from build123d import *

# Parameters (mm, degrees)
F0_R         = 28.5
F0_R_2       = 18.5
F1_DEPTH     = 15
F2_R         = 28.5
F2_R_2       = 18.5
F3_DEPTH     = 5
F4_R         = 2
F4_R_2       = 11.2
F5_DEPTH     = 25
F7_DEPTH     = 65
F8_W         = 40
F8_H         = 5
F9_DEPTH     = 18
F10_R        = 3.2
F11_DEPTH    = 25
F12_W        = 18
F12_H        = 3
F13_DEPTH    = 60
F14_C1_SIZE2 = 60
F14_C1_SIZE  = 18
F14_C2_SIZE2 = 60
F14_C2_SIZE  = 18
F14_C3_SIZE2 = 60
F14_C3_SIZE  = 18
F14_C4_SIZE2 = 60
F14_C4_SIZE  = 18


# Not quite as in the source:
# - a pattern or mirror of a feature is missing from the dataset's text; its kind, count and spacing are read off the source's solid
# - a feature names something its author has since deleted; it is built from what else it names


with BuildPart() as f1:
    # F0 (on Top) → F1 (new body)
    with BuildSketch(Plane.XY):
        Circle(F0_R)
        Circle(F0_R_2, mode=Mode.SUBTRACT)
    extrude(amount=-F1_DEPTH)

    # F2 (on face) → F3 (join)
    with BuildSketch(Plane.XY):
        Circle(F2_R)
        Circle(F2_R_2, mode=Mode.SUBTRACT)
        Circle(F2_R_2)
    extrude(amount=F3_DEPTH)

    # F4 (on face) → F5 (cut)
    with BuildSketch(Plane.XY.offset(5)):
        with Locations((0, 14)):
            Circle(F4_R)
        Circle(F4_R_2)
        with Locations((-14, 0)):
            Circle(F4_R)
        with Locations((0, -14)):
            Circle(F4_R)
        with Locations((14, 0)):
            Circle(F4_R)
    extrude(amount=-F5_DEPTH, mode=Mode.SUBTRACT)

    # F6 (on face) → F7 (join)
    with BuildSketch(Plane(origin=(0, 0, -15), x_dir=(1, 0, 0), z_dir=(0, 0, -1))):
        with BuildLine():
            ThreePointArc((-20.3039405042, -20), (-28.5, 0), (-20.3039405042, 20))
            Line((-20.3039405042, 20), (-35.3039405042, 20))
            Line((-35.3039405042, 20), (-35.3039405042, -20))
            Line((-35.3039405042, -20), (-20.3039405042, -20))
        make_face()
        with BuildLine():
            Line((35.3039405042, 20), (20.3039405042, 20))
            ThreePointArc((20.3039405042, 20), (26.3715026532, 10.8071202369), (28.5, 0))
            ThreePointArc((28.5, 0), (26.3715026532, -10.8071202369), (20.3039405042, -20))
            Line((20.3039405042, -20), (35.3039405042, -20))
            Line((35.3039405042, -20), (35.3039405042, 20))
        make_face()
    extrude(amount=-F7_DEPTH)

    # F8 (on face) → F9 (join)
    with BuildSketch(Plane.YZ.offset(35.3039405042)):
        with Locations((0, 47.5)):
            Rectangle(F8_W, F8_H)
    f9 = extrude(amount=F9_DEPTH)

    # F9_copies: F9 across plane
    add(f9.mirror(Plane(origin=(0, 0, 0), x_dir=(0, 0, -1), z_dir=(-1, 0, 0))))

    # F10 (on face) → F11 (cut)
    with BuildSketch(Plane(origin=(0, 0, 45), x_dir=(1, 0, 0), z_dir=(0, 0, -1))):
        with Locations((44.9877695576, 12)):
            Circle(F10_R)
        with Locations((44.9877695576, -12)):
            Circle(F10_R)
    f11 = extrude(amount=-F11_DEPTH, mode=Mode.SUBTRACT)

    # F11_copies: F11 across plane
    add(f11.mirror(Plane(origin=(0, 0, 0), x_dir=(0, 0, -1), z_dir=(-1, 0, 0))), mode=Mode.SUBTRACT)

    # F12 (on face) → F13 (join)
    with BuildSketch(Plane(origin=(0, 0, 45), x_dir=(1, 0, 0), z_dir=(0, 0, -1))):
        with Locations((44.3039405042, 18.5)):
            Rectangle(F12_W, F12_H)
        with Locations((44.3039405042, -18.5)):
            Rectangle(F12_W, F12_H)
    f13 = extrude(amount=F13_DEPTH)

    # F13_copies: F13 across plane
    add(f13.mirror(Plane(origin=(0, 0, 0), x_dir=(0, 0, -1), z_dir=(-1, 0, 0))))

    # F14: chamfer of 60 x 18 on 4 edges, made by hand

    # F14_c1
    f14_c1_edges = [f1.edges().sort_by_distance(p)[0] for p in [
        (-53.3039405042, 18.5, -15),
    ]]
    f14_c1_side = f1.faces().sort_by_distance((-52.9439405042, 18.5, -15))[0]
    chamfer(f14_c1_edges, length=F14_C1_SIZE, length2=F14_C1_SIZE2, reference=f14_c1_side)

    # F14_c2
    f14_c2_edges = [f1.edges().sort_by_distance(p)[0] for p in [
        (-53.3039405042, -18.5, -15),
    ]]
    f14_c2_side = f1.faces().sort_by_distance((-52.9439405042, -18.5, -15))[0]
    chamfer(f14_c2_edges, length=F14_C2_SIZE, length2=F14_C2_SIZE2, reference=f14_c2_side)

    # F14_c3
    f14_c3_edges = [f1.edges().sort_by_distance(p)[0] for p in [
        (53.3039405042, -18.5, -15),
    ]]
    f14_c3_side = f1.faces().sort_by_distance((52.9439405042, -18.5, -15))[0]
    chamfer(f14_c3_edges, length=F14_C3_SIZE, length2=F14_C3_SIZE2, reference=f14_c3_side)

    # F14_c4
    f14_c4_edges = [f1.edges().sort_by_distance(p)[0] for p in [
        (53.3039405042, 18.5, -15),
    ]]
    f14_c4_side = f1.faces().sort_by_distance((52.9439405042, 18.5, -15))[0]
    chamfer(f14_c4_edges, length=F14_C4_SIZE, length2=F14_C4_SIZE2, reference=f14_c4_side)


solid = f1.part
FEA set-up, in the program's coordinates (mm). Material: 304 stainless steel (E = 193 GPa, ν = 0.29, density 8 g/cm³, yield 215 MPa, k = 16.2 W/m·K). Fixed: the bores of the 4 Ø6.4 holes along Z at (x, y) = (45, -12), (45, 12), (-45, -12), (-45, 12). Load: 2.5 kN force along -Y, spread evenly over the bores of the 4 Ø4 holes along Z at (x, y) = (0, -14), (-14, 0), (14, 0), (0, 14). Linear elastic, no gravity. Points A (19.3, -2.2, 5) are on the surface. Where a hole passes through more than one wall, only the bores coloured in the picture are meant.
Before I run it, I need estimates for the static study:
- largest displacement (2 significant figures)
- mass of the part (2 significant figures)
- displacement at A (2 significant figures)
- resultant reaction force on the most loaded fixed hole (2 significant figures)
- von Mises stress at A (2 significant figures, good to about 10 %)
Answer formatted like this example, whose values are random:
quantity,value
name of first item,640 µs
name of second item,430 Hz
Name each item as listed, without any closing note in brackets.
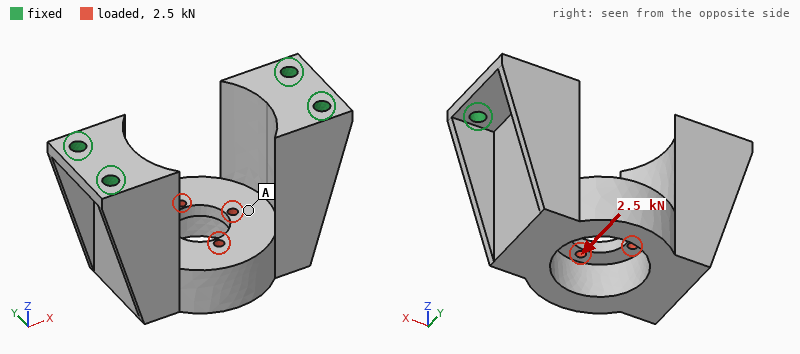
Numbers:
quantity,value
largest displacement,26 µm
mass of the part,760 g
displacement at A,18 µm
resultant reaction force on the most loaded fixed hole,2.1 kN
von Mises stress at A,11 MPa
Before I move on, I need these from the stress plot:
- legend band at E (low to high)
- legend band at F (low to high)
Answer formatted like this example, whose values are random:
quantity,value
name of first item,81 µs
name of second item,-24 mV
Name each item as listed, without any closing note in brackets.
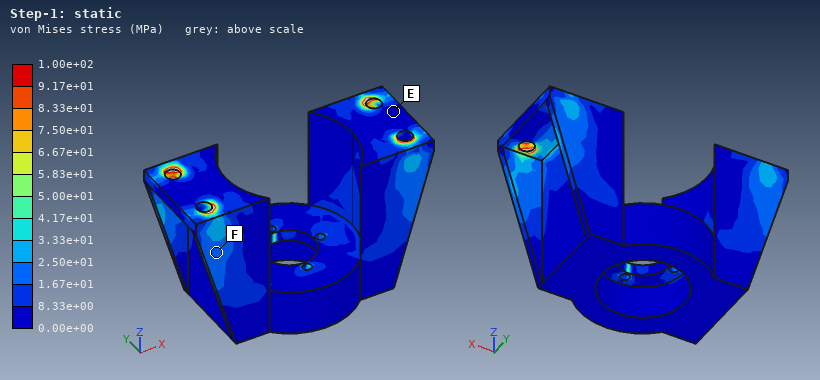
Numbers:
quantity,value
legend band at E,0.00e+00 to 8.33e+00 MPa
legend band at F,1.67e+01 to 2.50e+01 MPa
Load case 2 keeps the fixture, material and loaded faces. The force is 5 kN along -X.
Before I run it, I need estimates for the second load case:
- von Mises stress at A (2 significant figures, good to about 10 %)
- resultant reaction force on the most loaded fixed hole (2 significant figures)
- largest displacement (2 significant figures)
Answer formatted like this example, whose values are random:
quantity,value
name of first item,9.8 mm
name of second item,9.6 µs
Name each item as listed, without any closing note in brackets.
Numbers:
quantity,value
von Mises stress at A,25 MPa
resultant reaction force on the most loaded fixed hole,1.6 kN
largest displacement,41 µm
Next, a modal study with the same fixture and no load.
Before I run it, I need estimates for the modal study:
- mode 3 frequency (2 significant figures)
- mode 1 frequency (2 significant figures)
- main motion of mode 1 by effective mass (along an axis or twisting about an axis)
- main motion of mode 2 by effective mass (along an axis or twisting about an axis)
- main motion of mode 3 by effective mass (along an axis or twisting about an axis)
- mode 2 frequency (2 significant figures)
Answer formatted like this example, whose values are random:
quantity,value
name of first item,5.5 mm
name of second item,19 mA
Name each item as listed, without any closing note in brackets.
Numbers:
quantity,value
mode 3 frequency,3300 Hz
mode 1 frequency,2300 Hz
main motion of mode 1 by effective mass,along Y
main motion of mode 2 by effective mass,along X
main motion of mode 3 by effective mass,twisting about Z
mode 2 frequency,2600 Hz
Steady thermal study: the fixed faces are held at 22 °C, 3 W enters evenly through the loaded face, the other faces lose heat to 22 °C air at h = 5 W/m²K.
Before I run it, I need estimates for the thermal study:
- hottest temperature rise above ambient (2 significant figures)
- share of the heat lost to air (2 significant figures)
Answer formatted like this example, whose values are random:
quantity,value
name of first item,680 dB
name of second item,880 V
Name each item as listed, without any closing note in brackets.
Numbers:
quantity,value
hottest temperature rise above ambient,16 K
share of the heat lost to air,33 %
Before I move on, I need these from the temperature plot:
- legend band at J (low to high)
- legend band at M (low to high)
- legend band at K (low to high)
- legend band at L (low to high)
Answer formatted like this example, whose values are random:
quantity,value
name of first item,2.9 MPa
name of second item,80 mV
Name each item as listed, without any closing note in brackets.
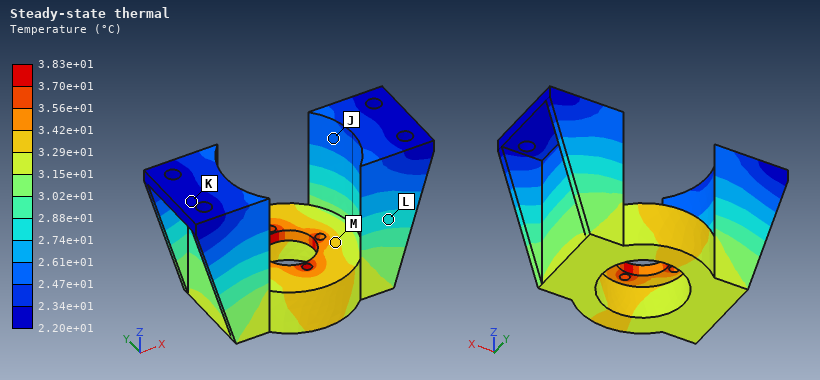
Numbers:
quantity,value
legend band at J,2.47e+01 to 2.61e+01 °C
legend band at M,3.29e+01 to 3.42e+01 °C
legend band at K,2.20e+01 to 2.34e+01 °C
legend band at L,2.74e+01 to 2.88e+01 °C
